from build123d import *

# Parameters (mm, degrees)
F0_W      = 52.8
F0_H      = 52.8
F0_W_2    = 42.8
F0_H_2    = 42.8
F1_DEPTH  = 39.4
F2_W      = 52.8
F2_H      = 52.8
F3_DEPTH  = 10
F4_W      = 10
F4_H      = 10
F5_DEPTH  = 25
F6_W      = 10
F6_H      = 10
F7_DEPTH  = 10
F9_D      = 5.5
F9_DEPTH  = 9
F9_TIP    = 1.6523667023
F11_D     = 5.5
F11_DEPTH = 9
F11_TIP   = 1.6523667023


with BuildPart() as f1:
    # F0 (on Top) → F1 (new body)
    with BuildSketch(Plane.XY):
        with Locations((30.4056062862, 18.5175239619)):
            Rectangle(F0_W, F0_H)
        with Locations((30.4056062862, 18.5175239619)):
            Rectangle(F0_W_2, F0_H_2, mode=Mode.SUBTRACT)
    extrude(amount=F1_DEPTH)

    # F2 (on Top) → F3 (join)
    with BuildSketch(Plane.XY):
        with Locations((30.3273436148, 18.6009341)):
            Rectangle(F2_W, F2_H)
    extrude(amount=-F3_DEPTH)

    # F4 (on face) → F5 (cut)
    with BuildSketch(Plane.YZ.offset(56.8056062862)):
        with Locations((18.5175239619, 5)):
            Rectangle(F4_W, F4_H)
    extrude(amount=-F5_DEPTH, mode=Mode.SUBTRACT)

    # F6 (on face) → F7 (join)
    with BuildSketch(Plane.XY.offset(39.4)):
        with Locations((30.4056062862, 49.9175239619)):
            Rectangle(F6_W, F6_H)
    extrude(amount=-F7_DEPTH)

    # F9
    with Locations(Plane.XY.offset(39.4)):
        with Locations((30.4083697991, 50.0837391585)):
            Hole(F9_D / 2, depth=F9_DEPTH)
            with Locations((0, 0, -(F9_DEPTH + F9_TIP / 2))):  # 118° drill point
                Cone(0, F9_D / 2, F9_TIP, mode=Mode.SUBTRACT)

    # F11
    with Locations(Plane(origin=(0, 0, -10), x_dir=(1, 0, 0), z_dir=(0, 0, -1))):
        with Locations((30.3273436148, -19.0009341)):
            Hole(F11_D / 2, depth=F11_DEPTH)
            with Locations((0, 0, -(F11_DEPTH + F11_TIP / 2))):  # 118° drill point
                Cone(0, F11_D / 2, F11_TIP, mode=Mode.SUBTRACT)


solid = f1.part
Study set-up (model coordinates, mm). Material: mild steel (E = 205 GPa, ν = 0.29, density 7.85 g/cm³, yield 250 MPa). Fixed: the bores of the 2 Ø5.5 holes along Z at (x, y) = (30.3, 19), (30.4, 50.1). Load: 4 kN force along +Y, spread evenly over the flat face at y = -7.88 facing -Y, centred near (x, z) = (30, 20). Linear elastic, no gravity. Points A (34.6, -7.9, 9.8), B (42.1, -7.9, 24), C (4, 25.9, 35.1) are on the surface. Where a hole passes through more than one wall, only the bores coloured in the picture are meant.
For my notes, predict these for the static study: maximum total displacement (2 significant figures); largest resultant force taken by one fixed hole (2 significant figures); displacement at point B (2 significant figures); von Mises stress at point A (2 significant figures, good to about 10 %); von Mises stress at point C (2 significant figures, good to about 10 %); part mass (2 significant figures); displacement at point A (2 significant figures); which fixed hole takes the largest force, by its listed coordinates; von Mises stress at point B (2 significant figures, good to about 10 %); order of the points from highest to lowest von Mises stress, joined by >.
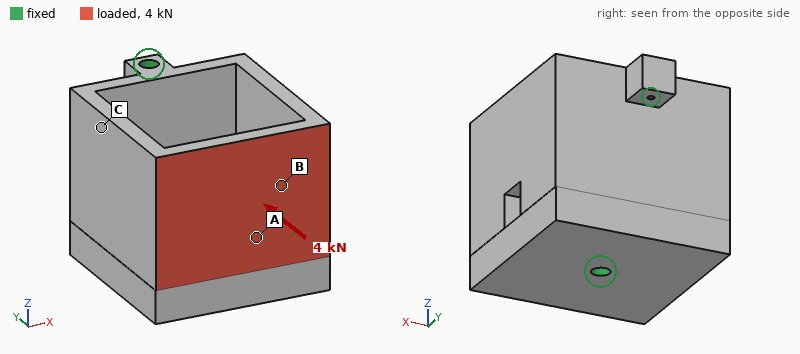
51 µm
3.8 kN
31 µm
21 MPa
8.6 MPa
510 g
23 µm
(30.3, 19)
32 MPa
B > A > C
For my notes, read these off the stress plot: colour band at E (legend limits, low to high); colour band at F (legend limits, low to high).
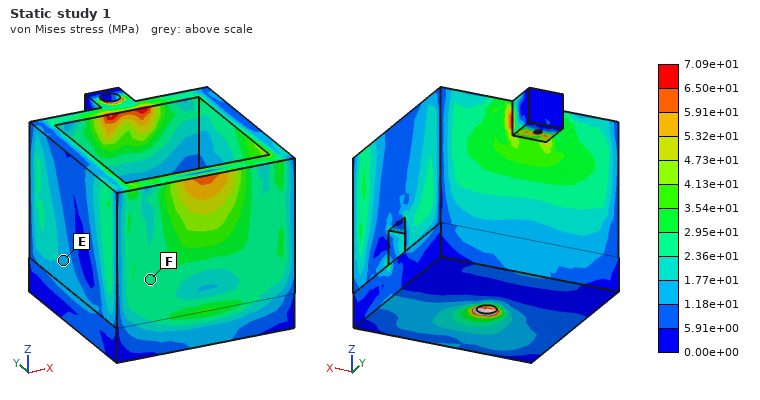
1.18e+01 to 1.77e+01 MPa
2.36e+01 to 2.95e+01 MPa
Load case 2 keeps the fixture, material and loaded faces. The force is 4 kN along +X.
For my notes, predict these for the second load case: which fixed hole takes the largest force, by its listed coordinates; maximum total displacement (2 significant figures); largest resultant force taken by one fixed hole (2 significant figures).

(30.3, 19)
0.12 mm
4.0 kN
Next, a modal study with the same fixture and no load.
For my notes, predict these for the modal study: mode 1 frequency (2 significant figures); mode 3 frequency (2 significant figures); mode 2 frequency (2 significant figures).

2400 Hz
4200 Hz
4000 Hz
